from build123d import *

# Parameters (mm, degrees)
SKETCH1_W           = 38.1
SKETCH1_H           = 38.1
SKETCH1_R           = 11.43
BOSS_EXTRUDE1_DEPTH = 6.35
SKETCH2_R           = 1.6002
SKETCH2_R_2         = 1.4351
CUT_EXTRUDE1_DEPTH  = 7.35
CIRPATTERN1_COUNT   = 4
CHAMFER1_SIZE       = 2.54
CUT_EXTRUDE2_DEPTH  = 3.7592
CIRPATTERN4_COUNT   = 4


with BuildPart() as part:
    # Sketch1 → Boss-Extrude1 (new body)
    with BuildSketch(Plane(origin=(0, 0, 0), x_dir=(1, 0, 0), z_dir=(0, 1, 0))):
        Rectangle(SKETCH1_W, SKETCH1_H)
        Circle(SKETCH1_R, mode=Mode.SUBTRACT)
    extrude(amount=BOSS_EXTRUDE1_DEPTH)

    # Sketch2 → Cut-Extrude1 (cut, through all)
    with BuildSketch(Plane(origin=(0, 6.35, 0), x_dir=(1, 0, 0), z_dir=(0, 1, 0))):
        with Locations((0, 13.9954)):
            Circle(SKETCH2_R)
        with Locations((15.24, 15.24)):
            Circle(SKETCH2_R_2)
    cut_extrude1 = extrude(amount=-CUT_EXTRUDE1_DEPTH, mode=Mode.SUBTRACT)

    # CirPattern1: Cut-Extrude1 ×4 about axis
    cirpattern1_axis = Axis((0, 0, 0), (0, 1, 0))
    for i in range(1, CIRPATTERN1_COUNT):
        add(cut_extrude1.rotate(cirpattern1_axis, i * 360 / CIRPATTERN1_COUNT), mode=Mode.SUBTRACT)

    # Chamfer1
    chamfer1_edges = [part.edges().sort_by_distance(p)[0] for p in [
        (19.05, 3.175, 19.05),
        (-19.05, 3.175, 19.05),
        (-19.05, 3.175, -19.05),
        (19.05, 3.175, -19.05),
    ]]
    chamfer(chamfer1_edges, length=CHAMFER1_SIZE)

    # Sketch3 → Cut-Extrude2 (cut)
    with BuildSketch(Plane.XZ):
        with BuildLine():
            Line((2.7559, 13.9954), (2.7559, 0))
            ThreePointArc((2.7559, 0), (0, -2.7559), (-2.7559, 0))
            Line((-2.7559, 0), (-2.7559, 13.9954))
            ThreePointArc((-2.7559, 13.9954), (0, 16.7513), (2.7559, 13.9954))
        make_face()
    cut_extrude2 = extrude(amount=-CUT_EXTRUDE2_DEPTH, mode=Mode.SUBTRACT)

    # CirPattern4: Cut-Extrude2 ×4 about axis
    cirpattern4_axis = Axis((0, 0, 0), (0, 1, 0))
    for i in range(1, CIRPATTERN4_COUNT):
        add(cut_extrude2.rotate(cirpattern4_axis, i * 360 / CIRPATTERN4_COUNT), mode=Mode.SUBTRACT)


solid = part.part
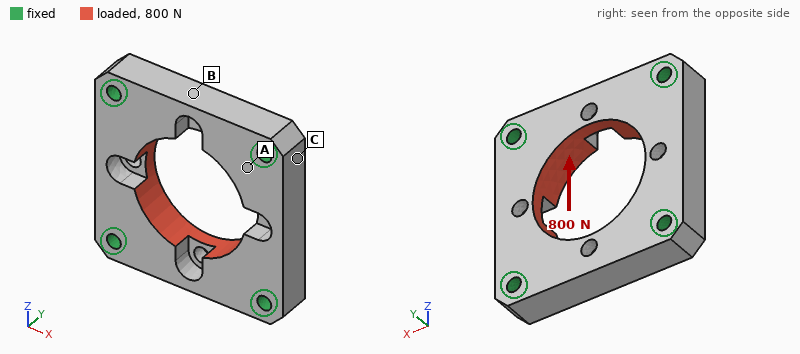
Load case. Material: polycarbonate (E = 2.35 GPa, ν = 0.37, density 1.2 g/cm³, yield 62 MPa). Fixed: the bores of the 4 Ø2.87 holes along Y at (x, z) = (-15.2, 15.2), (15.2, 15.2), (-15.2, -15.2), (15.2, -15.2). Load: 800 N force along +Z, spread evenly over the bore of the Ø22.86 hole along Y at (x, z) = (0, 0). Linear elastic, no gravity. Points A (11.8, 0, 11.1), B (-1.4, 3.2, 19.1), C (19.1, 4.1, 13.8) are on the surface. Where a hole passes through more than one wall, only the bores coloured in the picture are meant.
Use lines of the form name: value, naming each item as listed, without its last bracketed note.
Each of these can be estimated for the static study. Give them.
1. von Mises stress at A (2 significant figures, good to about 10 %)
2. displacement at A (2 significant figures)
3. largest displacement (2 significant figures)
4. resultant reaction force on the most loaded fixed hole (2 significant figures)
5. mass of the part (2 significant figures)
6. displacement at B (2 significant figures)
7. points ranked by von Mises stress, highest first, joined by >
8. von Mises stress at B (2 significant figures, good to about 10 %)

von Mises stress at A: 2.8 MPa
displacement at A: 19 µm
largest displacement: 69 µm
resultant reaction force on the most loaded fixed hole: 200 N
mass of the part: 7.1 g
displacement at B: 51 µm
points ranked by von Mises stress, highest first, joined by >: B > A > C
von Mises stress at B: 5.1 MPa
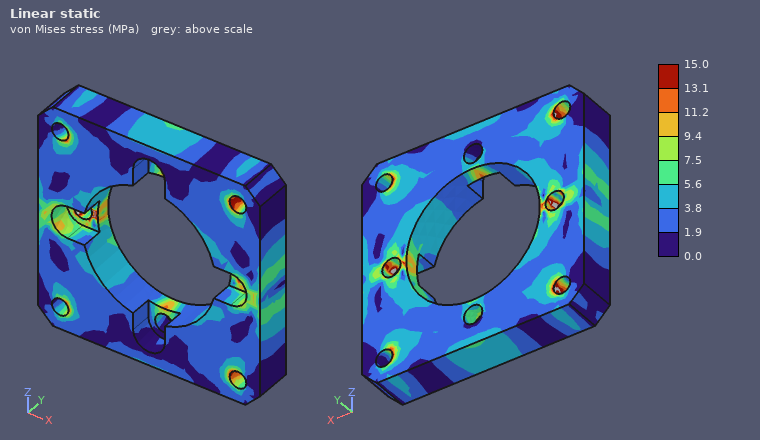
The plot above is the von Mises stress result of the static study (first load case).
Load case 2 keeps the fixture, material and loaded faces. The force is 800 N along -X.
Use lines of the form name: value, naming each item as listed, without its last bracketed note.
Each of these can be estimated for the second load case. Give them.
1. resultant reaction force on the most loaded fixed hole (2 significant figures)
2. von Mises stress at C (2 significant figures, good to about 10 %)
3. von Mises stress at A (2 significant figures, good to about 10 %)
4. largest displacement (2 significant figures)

resultant reaction force on the most loaded fixed hole: 200 N
von Mises stress at C: 4.2 MPa
von Mises stress at A: 2.7 MPa
largest displacement: 69 µm
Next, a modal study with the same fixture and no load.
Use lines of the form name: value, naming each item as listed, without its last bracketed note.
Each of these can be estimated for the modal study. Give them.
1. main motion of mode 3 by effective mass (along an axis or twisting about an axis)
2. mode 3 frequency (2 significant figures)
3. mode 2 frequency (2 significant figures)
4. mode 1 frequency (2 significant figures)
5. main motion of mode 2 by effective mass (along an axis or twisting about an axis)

main motion of mode 3 by effective mass: twisting about Z
mode 3 frequency: 8100 Hz
mode 2 frequency: 7700 Hz
mode 1 frequency: 6400 Hz
main motion of mode 2 by effective mass: along Y
